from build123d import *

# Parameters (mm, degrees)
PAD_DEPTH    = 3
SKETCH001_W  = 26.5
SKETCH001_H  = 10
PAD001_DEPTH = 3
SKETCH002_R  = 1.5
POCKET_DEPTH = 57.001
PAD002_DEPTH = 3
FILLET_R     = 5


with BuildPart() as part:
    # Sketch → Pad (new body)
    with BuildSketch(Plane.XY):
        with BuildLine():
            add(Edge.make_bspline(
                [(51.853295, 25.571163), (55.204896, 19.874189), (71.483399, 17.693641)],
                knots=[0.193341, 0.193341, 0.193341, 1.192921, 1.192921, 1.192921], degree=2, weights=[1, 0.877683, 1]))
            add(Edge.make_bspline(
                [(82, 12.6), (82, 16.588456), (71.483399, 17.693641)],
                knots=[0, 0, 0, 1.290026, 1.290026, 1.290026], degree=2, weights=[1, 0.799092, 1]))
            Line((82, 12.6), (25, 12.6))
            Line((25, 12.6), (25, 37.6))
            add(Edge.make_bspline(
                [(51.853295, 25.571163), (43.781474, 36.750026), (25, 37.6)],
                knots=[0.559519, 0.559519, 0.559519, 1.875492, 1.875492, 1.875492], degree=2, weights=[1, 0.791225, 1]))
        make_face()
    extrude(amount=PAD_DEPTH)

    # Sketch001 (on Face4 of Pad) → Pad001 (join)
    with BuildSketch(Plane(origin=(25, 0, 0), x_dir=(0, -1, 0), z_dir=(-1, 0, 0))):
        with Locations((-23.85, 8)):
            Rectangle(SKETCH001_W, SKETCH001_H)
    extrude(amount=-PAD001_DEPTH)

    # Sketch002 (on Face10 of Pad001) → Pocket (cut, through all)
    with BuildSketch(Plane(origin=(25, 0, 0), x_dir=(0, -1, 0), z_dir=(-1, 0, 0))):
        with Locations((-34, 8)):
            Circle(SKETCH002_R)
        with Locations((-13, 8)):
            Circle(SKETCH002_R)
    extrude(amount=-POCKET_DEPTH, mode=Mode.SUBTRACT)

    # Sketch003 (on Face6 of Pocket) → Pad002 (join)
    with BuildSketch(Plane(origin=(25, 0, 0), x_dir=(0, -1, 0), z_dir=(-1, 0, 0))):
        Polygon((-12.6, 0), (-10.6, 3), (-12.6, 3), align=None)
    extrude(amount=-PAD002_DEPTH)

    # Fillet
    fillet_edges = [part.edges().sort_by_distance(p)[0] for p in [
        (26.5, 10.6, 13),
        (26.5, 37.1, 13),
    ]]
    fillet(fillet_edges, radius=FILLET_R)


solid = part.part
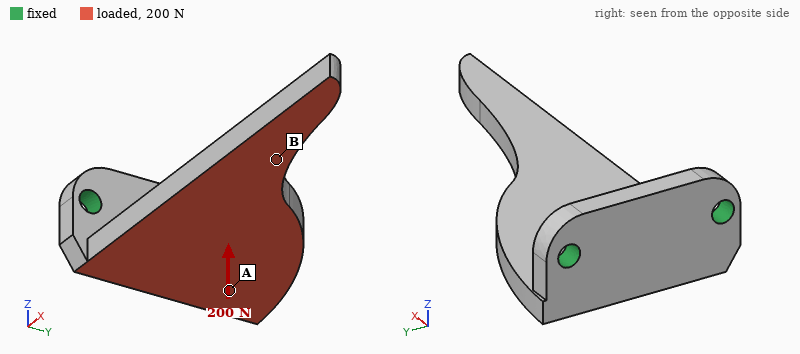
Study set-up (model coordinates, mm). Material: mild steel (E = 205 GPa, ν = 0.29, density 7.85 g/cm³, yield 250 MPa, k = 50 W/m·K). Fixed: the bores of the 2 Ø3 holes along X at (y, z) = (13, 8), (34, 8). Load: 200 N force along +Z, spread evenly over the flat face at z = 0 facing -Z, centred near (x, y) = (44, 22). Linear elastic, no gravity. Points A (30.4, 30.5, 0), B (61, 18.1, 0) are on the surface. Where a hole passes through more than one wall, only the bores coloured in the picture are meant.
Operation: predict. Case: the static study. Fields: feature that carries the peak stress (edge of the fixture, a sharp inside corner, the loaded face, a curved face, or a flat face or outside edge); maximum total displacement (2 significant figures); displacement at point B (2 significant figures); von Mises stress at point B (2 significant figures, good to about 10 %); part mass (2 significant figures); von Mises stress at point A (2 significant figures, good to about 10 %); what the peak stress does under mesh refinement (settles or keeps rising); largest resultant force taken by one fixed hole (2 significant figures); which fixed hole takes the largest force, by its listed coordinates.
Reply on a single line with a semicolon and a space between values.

edge of the fixture; 0.34 mm; 0.17 mm; 23 MPa; 24 g; 66 MPa; keeps rising; 120 N; (13, 8)
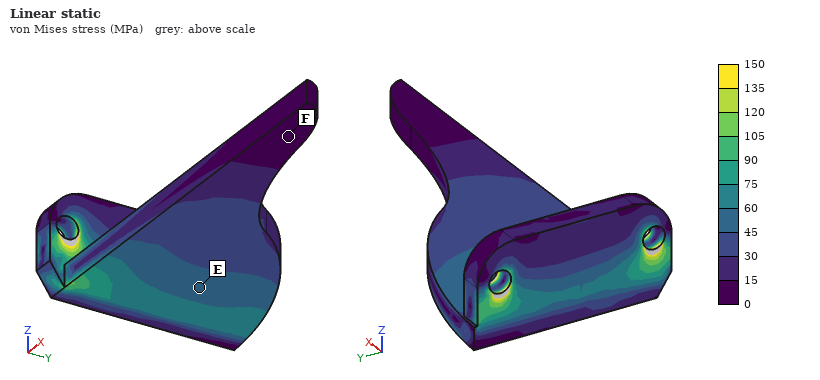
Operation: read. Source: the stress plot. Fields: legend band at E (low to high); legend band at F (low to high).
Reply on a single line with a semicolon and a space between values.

45 to 60 MPa; 0 to 15 MPa
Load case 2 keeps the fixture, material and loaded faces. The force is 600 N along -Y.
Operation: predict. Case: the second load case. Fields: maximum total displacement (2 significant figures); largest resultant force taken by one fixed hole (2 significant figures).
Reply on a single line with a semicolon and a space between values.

63 µm; 620 N
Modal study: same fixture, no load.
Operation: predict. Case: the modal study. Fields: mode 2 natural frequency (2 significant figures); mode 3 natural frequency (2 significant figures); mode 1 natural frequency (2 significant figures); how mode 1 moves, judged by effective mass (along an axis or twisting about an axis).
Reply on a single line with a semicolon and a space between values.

5000 Hz; 5200 Hz; 1300 Hz; along Z
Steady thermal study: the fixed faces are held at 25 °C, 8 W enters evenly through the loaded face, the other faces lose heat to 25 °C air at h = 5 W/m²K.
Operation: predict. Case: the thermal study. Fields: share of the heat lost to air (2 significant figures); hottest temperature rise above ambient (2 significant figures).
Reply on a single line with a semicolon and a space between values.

3.2 %; 71 K
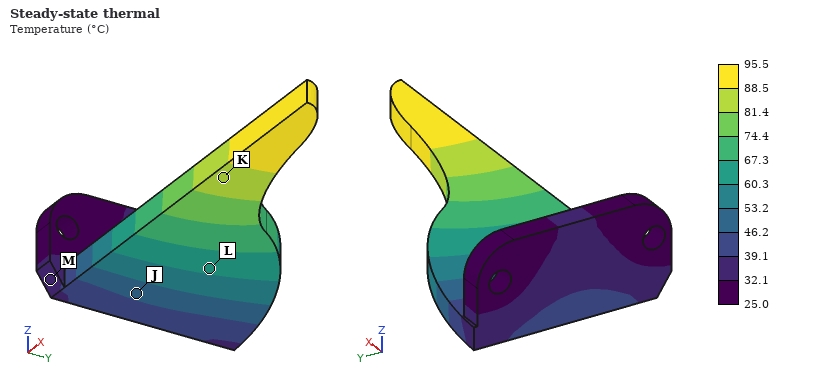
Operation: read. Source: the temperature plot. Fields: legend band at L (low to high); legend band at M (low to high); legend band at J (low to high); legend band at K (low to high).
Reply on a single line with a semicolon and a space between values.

60.3 to 67.3 °C; 32.1 to 39.1 °C; 46.2 to 53.2 °C; 81.4 to 88.5 °C
